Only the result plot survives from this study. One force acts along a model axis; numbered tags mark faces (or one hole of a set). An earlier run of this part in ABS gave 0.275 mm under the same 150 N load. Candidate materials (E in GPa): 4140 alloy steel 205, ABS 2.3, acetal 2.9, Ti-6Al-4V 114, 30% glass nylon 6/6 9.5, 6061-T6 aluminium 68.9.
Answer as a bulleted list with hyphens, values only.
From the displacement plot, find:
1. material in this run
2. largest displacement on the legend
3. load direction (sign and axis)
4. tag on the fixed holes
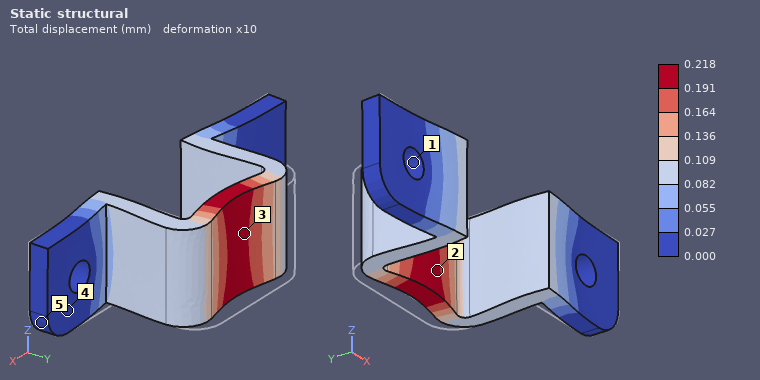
- acetal
- 0.218 mm
- -Y
- 1
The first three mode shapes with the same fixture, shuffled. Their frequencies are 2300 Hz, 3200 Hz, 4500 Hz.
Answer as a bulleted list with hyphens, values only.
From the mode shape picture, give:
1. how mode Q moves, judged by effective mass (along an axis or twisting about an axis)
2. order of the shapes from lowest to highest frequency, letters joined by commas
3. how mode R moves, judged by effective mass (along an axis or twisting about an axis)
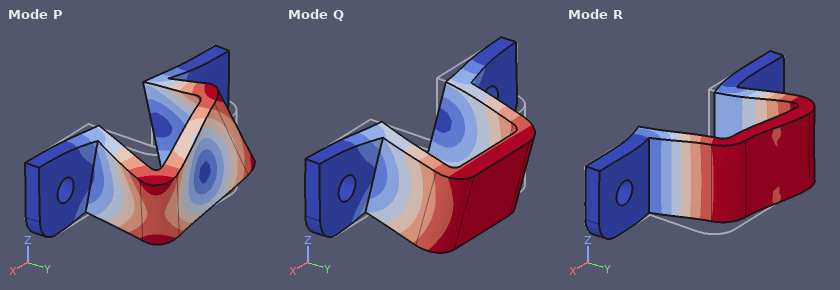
- along Z
- Q, R, P
- along X
